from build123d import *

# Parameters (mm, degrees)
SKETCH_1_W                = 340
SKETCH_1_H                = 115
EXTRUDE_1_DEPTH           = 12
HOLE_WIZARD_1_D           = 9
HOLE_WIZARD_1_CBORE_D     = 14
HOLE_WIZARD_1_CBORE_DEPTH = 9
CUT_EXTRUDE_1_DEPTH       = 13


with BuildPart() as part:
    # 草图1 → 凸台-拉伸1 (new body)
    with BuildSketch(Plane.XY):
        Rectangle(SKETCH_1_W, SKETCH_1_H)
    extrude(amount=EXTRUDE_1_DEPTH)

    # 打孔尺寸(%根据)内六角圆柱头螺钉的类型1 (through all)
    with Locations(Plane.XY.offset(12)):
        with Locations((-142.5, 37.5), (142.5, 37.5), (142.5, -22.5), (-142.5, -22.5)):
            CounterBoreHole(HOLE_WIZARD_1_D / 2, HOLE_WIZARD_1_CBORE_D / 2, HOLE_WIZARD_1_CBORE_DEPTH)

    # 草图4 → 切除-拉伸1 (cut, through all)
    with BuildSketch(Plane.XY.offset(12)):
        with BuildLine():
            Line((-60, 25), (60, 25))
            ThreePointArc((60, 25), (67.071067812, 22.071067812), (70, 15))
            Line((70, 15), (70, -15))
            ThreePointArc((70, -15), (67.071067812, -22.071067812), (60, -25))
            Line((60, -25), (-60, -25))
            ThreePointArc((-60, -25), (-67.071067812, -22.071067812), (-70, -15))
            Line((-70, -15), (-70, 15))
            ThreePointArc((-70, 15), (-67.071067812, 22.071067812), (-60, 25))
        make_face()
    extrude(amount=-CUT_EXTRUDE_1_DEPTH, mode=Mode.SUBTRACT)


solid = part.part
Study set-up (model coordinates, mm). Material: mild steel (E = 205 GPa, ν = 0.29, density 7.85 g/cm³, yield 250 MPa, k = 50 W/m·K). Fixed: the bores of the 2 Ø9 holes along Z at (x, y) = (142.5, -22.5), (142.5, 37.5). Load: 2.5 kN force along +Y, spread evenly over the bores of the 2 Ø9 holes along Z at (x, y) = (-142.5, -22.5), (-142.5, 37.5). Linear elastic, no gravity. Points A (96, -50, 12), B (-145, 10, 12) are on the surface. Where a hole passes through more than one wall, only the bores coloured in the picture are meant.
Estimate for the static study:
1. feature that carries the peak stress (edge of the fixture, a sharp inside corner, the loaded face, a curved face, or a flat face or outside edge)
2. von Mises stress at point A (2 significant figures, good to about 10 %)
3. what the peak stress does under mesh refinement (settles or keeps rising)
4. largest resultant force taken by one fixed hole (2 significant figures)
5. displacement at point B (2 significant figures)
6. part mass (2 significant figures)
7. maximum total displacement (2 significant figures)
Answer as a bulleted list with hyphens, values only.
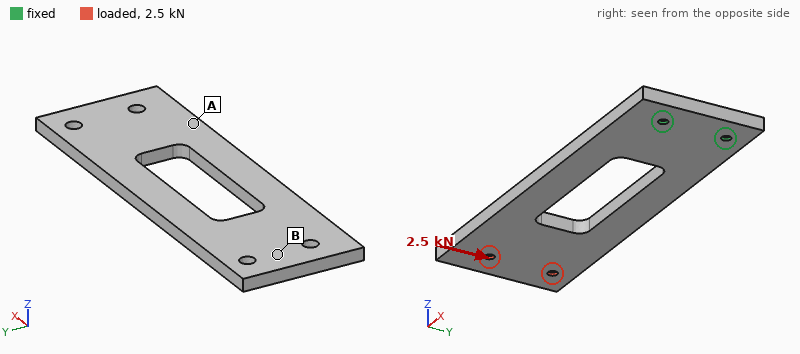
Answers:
- edge of the fixture
- 25 MPa
- keeps rising
- 11 kN
- 0.20 mm
- 3.0 kg
- 0.25 mm
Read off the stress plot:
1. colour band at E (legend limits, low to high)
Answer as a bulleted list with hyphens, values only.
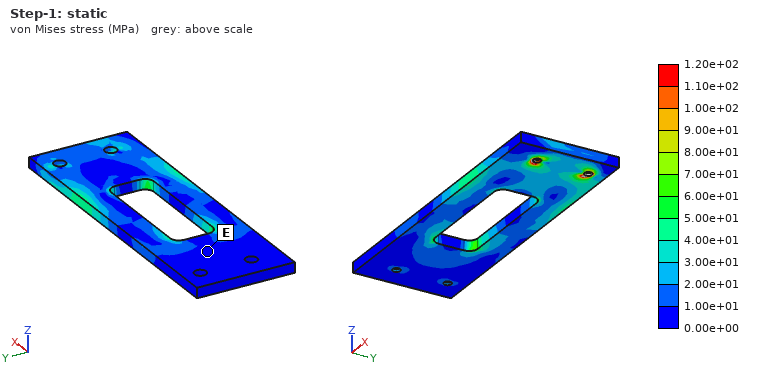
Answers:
- 0.00e+00 to 1.00e+01 MPa
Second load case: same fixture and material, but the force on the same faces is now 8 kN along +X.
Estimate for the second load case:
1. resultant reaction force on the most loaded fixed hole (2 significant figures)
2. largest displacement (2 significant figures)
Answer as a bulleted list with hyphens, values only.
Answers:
- 4.0 kN
- 0.70 mm
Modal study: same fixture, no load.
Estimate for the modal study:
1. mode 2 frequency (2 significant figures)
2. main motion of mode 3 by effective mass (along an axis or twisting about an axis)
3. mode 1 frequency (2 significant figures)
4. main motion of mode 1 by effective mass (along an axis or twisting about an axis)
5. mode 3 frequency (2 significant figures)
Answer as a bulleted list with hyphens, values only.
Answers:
- 430 Hz
- along Z
- 73 Hz
- along Z
- 510 Hz
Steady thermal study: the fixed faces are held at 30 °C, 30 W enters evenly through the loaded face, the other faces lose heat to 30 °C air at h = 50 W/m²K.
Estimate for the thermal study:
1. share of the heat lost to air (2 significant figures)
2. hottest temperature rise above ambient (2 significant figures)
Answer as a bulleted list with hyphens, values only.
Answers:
- 99 %
- 37 K
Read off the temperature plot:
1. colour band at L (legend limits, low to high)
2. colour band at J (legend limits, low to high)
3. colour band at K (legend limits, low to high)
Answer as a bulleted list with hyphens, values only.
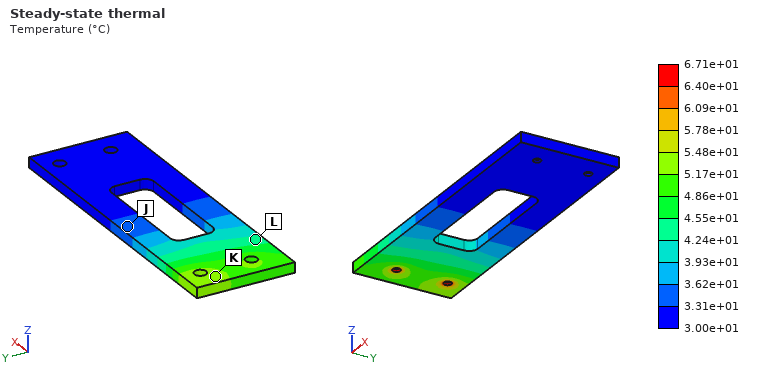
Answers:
- 4.24e+01 to 4.55e+01 °C
- 3.31e+01 to 3.62e+01 °C
- 5.17e+01 to 5.48e+01 °C
